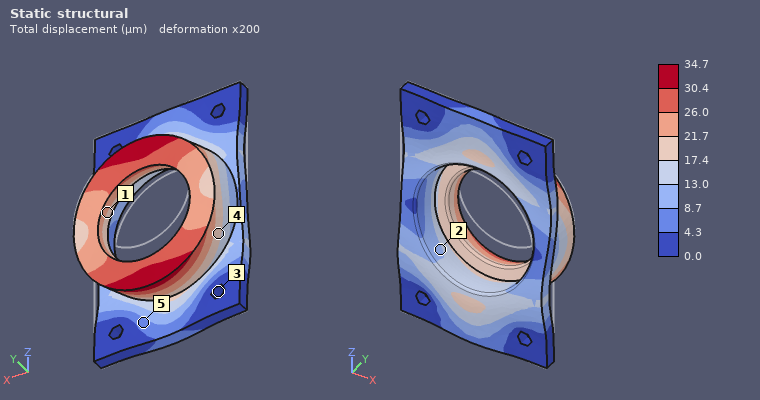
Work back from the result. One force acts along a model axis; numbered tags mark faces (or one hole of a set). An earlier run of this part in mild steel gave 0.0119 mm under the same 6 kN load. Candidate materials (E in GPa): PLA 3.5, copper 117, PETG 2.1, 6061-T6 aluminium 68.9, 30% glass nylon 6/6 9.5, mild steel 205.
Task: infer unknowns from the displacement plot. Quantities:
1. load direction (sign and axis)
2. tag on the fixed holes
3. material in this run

-Z
3
6061-T6 aluminium
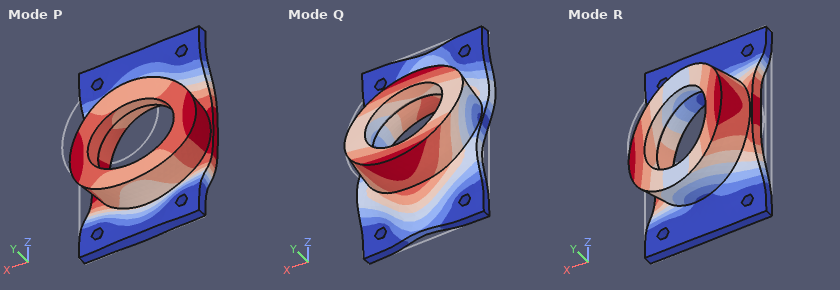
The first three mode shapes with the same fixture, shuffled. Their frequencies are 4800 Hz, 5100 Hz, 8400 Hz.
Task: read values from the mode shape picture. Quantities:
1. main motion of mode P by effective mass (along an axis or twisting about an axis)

along Y
